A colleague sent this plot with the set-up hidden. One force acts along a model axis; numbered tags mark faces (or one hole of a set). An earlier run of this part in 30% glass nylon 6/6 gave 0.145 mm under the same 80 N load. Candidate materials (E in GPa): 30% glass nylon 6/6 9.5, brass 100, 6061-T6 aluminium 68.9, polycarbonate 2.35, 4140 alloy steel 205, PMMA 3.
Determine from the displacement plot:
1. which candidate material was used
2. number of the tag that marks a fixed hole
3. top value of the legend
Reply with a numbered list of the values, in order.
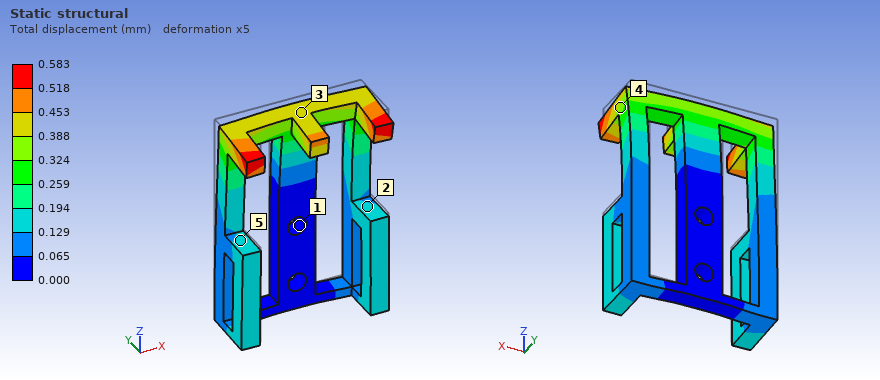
1. polycarbonate
2. 1
3. 0.583 mm
